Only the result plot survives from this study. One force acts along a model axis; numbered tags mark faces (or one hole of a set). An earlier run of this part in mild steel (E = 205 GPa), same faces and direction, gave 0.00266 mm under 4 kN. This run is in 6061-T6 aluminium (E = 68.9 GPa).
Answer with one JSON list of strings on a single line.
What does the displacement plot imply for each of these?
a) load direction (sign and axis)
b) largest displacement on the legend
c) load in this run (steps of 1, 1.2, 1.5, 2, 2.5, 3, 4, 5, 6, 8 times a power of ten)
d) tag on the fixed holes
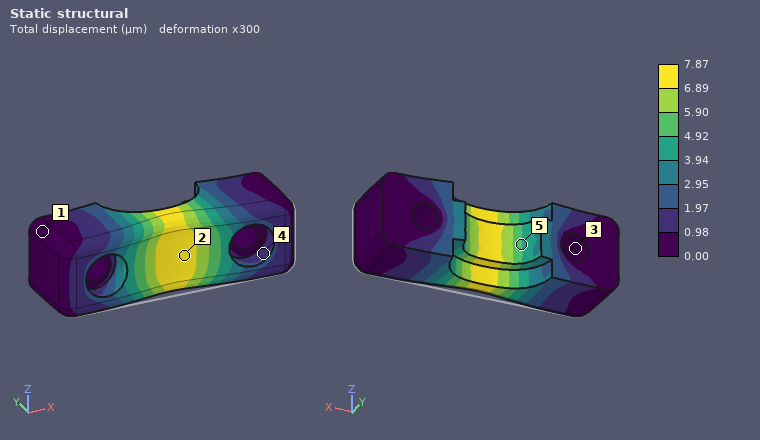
["+Y", "7.87 µm", "4 kN", "3"]
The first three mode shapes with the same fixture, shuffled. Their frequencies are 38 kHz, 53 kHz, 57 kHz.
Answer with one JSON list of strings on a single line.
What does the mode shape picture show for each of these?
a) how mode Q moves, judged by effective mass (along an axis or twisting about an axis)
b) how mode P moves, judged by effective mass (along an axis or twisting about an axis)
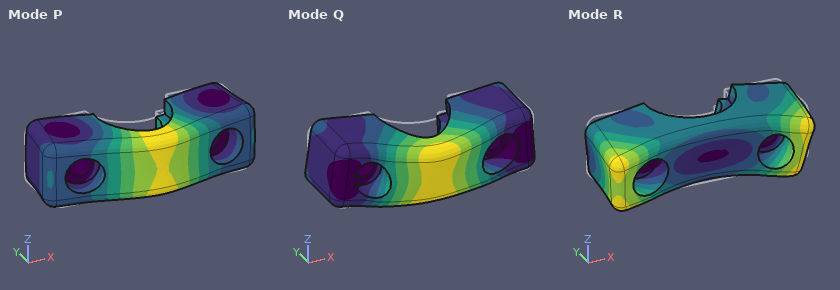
["along Z", "along Y"]
